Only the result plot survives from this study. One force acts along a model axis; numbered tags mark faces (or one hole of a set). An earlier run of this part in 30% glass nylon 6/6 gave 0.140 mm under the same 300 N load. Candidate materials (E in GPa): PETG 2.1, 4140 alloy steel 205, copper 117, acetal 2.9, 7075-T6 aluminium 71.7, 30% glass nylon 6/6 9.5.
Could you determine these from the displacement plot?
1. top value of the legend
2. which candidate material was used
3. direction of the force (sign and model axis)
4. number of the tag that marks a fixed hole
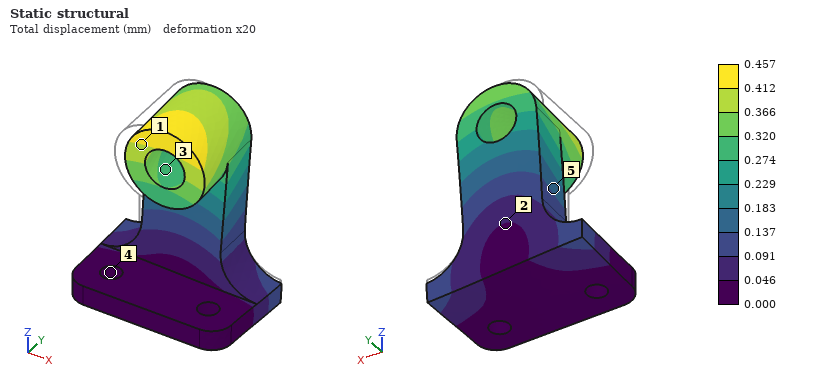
0.457 mm
acetal
+X
4
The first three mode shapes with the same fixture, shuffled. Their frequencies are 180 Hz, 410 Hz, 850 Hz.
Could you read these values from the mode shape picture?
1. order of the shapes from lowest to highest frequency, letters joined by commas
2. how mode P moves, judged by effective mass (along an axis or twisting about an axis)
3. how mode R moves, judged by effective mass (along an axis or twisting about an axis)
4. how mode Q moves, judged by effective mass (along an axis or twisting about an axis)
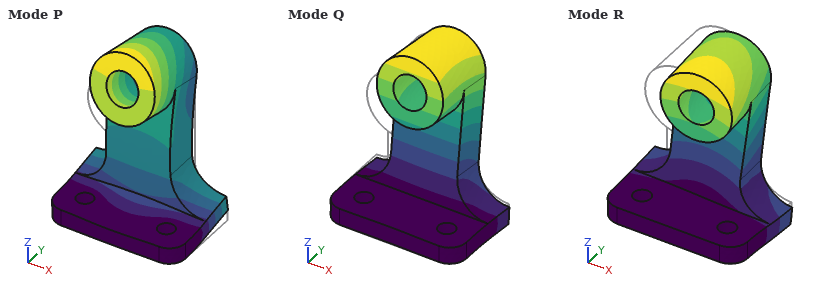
Q, R, P
along Z
along X
along Y
